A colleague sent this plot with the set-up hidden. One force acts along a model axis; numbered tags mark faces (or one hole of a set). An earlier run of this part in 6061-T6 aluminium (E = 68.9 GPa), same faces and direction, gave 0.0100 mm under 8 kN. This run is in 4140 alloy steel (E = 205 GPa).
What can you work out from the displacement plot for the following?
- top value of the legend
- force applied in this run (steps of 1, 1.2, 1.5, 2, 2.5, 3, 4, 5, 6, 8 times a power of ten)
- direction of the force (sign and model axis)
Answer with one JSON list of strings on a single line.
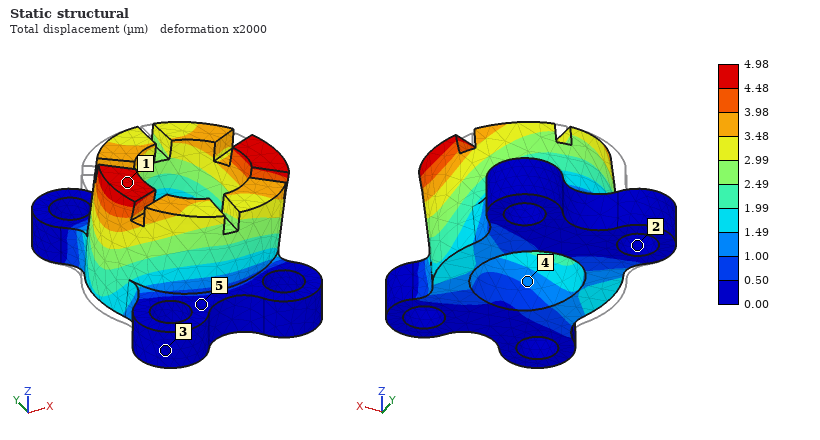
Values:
["4.98 µm", "12 kN", "+X"]
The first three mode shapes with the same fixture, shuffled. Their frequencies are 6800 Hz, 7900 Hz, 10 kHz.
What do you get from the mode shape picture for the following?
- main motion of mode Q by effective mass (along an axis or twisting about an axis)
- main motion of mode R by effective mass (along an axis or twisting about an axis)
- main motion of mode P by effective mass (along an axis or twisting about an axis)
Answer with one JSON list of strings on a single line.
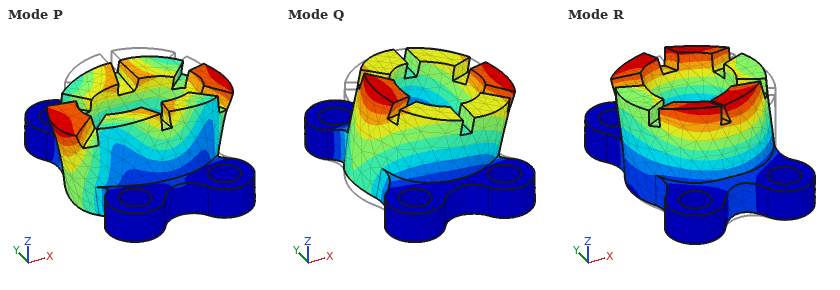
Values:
["along X", "along Y", "along Z"]
